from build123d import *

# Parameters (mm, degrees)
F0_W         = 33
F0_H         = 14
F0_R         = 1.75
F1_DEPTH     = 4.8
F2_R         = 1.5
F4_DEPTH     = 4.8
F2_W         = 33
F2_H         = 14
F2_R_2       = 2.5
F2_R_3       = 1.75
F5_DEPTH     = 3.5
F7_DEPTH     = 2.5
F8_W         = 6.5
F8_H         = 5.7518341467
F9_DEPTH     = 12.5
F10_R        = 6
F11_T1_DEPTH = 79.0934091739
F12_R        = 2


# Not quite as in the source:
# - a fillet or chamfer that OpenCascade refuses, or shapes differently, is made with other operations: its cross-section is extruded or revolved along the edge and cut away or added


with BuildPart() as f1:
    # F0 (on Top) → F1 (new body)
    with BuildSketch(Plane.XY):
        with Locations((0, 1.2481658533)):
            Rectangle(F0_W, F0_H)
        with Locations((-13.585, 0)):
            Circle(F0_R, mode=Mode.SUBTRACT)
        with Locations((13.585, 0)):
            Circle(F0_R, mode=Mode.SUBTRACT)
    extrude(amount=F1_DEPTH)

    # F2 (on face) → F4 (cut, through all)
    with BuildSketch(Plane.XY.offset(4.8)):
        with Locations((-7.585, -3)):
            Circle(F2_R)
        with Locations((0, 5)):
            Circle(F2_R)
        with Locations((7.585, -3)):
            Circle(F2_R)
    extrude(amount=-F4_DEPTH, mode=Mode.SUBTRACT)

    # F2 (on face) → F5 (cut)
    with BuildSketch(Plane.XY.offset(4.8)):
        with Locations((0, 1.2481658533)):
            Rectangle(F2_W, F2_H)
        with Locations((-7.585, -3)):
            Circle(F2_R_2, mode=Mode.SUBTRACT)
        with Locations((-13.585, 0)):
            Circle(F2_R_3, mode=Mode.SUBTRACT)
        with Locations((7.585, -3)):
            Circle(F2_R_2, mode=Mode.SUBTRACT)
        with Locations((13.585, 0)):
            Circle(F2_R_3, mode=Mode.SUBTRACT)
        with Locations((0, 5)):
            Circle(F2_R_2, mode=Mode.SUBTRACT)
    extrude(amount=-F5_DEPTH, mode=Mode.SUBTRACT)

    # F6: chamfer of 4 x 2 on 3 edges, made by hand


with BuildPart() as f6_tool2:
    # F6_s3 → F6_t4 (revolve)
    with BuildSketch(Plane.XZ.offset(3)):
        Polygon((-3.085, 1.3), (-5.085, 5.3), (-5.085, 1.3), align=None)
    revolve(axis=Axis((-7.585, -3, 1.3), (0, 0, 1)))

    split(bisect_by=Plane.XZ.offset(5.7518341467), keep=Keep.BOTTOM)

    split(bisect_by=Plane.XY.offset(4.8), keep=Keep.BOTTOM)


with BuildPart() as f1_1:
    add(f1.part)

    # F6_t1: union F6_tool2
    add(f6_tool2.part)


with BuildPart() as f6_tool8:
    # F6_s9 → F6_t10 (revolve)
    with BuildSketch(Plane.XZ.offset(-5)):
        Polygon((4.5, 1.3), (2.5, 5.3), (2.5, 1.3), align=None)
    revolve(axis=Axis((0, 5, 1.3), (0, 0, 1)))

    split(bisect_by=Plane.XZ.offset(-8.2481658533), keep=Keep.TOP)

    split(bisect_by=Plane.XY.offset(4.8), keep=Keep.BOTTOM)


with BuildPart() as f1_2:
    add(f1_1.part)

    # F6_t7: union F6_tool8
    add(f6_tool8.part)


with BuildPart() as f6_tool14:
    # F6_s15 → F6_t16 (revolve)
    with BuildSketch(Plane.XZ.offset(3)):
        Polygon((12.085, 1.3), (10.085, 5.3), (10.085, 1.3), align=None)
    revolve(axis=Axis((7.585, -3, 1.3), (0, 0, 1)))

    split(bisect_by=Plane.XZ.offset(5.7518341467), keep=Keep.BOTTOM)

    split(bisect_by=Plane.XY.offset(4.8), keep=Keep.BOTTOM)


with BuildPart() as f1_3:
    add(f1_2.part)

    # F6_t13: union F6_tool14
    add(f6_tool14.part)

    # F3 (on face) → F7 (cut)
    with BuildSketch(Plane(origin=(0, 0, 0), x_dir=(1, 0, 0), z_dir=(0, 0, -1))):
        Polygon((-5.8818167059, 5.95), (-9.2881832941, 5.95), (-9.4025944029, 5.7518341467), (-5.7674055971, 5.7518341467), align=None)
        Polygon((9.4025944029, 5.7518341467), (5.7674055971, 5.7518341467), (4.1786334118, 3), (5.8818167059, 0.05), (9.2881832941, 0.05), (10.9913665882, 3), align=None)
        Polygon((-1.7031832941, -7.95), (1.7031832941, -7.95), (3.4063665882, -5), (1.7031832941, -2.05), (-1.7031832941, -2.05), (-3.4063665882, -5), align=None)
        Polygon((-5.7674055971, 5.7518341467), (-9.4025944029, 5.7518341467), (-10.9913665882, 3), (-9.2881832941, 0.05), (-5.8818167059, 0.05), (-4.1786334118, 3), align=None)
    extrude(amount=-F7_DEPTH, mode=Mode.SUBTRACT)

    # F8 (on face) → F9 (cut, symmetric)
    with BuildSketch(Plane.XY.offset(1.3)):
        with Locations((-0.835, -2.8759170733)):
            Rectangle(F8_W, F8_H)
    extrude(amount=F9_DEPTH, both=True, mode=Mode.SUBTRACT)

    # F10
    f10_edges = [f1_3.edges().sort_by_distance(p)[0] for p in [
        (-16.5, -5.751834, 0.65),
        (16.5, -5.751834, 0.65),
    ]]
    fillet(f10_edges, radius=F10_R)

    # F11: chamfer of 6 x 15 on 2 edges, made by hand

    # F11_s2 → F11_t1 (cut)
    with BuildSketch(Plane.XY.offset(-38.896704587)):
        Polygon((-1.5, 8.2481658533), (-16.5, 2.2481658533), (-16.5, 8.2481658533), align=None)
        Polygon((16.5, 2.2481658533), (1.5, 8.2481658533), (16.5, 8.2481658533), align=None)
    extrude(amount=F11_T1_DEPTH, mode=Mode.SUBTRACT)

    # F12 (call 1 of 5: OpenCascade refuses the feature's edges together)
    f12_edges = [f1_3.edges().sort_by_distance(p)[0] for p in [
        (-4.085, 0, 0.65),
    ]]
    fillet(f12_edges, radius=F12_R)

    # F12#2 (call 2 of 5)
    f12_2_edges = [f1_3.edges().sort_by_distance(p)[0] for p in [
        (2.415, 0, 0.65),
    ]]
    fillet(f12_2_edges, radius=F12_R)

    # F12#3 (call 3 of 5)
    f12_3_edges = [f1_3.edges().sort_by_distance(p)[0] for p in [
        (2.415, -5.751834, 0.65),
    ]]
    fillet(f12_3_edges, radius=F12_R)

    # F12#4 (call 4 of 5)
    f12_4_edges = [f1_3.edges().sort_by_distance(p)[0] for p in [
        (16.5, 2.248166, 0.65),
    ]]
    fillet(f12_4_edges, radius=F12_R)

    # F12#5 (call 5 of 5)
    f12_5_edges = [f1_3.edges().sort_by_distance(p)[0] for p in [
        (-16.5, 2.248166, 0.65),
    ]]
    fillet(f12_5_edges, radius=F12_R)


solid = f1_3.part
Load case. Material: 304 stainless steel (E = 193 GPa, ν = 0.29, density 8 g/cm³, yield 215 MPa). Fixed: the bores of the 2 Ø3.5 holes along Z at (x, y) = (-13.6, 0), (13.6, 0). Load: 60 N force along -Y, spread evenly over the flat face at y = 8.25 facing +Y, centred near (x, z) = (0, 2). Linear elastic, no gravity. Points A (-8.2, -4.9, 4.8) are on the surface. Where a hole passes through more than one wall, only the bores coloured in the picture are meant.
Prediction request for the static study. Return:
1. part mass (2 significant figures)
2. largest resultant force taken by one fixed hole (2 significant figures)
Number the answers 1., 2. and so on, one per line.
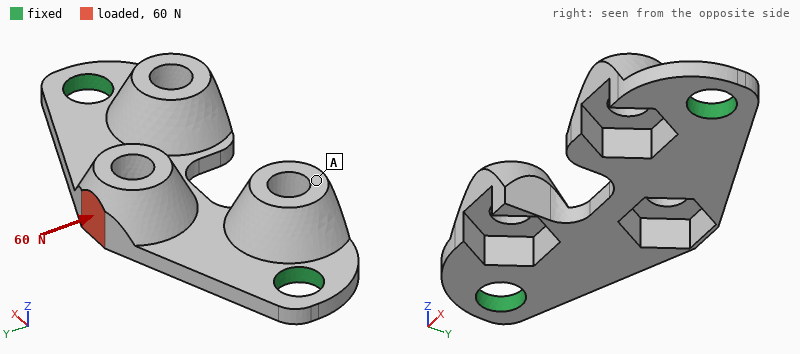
1. 4.2 g
2. 36 N
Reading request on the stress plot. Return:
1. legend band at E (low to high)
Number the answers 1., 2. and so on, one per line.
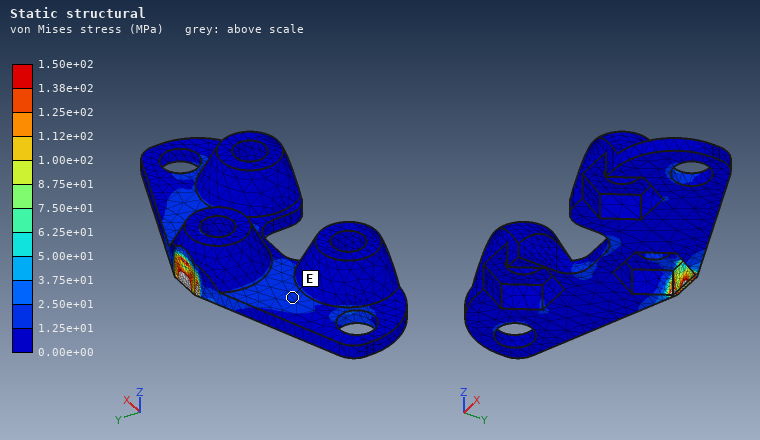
1. 1.25e+01 to 2.50e+01 MPa
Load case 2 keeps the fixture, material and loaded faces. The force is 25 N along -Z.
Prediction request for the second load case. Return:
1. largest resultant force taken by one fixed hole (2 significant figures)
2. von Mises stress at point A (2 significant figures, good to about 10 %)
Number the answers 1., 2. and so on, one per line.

1. 19 N
2. 5.0 MPa
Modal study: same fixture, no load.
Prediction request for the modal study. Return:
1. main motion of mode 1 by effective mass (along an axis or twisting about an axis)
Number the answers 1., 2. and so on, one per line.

1. along Z
